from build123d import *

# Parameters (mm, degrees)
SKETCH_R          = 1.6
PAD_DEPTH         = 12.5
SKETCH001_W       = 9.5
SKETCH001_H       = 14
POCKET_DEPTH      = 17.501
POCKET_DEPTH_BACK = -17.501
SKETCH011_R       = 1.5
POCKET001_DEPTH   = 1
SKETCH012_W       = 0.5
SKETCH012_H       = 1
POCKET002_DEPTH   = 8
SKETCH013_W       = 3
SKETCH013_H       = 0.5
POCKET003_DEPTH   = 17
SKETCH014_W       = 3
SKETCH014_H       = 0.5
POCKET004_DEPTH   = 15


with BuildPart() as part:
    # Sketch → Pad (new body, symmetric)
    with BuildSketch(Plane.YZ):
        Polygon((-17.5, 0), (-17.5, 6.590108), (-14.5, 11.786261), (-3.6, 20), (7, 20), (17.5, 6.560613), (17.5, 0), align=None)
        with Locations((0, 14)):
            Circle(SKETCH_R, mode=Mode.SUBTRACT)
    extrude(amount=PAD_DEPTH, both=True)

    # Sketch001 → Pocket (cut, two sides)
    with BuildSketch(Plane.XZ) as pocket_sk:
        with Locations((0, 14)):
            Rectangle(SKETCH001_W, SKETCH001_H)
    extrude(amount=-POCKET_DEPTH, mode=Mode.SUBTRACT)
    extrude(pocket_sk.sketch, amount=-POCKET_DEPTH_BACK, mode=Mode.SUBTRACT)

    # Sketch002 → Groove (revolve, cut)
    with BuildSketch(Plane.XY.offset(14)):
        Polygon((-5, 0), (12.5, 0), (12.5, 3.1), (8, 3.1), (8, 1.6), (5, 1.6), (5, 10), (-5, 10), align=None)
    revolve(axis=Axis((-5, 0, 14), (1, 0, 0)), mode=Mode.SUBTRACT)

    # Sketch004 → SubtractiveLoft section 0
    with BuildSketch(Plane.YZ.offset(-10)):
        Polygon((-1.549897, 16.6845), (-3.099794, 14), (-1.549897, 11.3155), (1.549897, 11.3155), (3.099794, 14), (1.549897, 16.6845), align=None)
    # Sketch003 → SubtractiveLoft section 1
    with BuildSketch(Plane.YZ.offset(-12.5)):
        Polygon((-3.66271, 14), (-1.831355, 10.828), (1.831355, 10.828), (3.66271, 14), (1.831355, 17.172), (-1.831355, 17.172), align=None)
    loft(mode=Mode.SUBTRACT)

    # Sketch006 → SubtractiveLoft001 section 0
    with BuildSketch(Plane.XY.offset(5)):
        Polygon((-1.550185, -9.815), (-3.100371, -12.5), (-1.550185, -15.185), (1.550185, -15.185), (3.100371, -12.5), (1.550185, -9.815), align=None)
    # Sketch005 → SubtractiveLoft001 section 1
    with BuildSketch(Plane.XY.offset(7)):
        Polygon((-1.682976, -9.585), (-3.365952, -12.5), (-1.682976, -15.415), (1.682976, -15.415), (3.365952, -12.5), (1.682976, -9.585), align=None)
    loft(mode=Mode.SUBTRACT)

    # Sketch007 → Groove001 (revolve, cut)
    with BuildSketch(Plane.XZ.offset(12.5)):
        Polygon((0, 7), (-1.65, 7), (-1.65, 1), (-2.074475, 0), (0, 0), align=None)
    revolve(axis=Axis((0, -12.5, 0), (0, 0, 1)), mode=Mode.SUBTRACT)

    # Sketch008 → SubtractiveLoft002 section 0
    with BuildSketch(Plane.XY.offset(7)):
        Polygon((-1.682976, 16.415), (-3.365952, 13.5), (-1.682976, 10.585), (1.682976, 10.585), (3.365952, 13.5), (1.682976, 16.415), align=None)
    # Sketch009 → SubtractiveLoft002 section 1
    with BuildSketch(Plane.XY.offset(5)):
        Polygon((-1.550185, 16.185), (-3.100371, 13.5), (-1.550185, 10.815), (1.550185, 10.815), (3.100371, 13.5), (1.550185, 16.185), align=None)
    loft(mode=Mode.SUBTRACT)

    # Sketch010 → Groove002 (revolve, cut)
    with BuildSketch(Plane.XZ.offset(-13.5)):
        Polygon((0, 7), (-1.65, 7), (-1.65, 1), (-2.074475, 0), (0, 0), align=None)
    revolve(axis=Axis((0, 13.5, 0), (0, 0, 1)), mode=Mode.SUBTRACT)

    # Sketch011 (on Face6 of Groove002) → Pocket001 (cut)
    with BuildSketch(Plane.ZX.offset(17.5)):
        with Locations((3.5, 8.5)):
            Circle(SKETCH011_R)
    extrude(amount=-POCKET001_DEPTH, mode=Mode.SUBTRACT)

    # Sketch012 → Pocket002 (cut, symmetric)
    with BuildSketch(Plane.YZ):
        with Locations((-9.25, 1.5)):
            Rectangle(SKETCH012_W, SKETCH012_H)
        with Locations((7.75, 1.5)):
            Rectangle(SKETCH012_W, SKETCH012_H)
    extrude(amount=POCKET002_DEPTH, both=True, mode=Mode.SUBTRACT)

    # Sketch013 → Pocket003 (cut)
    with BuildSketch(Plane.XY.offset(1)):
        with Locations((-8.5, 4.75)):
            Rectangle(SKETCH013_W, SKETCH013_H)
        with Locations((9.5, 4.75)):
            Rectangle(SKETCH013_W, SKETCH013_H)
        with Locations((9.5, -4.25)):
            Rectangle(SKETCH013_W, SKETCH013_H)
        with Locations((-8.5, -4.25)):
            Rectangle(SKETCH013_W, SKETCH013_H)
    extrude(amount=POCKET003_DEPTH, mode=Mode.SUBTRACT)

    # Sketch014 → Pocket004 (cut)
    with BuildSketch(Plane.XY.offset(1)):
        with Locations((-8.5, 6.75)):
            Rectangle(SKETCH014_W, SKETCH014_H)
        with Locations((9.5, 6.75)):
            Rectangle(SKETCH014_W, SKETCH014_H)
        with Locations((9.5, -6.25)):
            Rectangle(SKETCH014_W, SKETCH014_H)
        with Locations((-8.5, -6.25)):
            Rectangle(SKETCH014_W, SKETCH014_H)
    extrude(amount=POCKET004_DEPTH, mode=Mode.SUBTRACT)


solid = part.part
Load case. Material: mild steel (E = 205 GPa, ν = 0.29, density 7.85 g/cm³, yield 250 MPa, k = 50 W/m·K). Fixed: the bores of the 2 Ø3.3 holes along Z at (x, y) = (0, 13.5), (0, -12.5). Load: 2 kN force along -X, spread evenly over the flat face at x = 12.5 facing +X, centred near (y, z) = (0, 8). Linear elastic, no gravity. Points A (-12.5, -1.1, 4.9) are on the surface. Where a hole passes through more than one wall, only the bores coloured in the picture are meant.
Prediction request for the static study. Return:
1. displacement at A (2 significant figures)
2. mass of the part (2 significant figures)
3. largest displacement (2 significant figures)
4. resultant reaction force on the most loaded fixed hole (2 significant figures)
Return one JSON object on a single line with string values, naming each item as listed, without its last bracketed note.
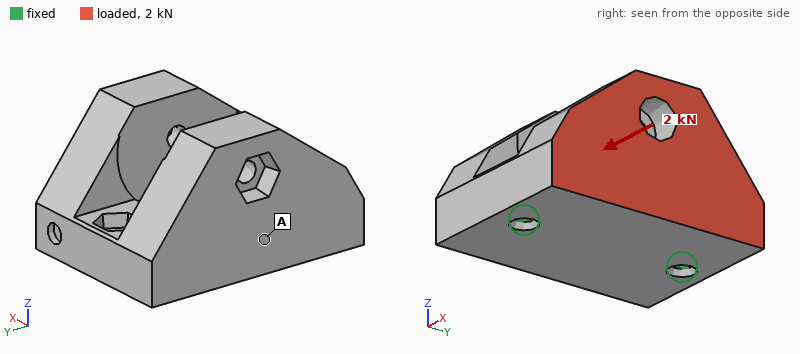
{"displacement at A": "4.6 µm", "mass of the part": "77 g", "largest displacement": "22 µm", "resultant reaction force on the most loaded fixed hole": "1.0 kN"}
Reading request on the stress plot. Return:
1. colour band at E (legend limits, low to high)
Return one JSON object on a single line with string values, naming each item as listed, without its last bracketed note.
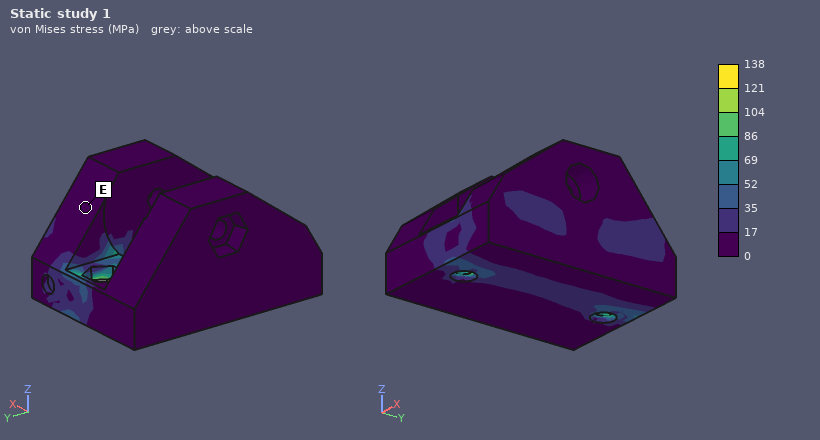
{"colour band at E": "0 to 17 MPa"}
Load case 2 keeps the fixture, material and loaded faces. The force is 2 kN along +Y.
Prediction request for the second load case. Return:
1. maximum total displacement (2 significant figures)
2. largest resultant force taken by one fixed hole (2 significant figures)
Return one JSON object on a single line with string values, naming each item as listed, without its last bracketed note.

{"maximum total displacement": "3.7 µm", "largest resultant force taken by one fixed hole": "1.4 kN"}
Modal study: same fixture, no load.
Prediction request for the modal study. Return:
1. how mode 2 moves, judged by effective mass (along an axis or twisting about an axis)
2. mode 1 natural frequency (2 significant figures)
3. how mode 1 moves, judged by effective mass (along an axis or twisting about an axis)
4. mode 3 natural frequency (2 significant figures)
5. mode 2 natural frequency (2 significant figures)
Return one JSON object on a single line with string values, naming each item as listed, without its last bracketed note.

{"how mode 2 moves, judged by effective mass": "along Z", "mode 1 natural frequency": "7500 Hz", "how mode 1 moves, judged by effective mass": "along X", "mode 3 natural frequency": "20 kHz", "mode 2 natural frequency": "12 kHz"}
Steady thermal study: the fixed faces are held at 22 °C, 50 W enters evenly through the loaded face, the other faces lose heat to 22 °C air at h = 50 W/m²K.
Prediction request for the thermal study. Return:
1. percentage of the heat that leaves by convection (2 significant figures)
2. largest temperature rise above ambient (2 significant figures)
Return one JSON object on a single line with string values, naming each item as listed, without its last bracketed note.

{"percentage of the heat that leaves by convection": "13 %", "largest temperature rise above ambient": "71 K"}
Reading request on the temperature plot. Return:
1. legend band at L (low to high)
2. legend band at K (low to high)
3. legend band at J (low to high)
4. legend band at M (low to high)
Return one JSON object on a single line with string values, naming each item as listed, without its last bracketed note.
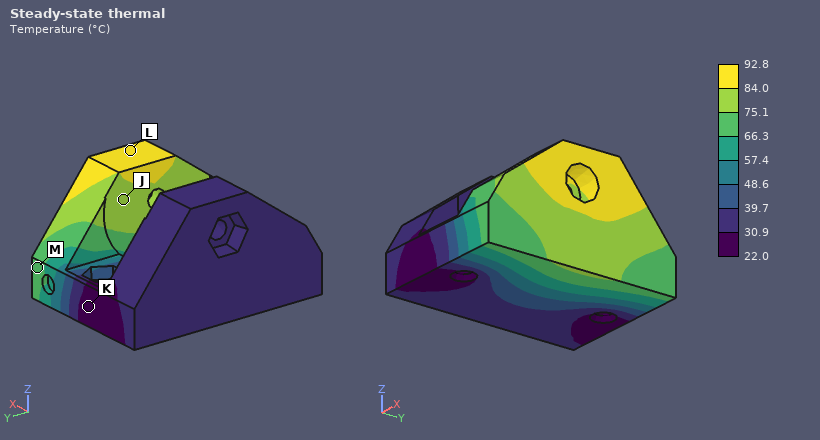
{"legend band at L": "84.0 to 92.8 °C", "legend band at K": "22.0 to 30.9 °C", "legend band at J": "75.1 to 84.0 °C", "legend band at M": "66.3 to 75.1 °C"}
